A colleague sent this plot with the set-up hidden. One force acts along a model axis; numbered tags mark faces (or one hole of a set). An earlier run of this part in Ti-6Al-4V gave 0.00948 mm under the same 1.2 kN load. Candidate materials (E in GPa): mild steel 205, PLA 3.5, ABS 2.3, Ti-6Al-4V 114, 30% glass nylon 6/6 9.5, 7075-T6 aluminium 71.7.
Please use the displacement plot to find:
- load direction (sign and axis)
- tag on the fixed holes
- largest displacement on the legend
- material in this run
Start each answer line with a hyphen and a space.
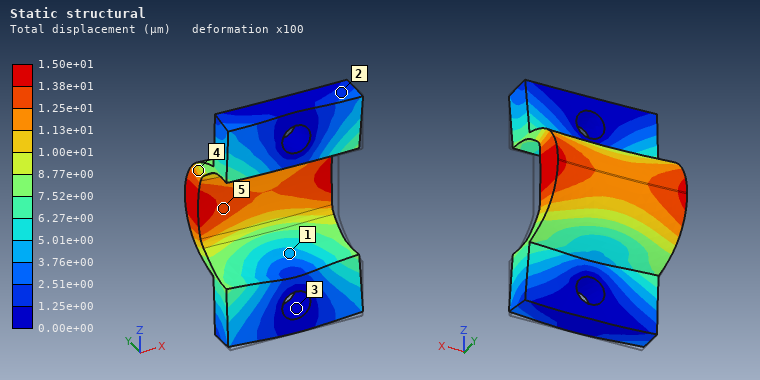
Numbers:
- +Y
- 3
- 1.50e+01 µm
- 7075-T6 aluminium
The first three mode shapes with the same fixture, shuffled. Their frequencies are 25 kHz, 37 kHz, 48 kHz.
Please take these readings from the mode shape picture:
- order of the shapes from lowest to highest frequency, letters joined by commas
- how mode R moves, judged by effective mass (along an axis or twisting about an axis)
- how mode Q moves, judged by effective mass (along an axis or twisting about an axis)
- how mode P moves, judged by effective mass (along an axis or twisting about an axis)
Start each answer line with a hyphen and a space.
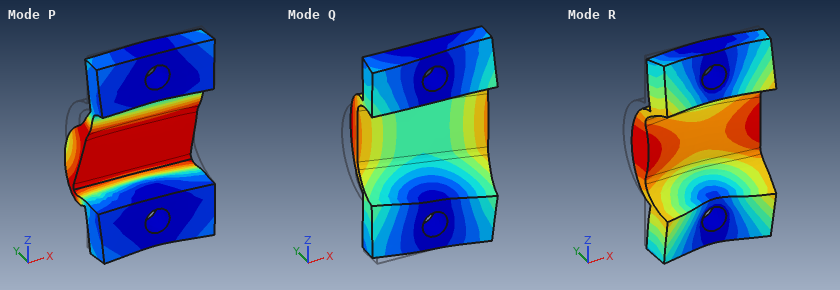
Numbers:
- Q, P, R
- along Y
- along X
- along Z
